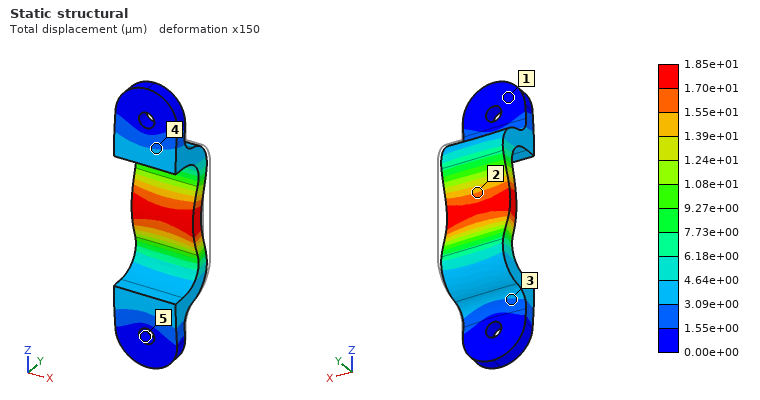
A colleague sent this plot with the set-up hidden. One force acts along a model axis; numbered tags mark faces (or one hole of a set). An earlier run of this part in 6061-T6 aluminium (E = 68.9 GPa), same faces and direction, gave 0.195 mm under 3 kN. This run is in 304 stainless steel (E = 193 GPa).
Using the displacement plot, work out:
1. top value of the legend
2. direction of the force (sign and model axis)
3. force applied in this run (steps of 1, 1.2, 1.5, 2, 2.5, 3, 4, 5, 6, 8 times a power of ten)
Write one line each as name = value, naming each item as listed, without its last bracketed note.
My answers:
top value of the legend = 1.85e+01 µm
direction of the force = -Y
force applied in this run = 800 N
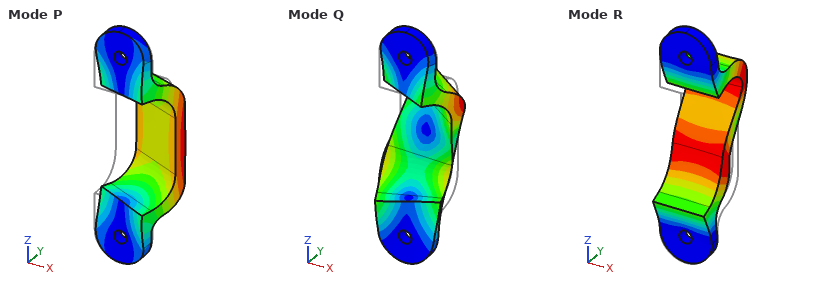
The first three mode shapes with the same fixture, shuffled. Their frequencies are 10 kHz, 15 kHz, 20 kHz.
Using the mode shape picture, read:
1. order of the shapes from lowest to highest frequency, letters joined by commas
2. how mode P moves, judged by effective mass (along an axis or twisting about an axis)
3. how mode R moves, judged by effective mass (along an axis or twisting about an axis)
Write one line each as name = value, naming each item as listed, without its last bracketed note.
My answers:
order of the shapes from lowest to highest frequency, letters joined by commas = P, R, Q
how mode P moves, judged by effective mass = along X
how mode R moves, judged by effective mass = along Z
